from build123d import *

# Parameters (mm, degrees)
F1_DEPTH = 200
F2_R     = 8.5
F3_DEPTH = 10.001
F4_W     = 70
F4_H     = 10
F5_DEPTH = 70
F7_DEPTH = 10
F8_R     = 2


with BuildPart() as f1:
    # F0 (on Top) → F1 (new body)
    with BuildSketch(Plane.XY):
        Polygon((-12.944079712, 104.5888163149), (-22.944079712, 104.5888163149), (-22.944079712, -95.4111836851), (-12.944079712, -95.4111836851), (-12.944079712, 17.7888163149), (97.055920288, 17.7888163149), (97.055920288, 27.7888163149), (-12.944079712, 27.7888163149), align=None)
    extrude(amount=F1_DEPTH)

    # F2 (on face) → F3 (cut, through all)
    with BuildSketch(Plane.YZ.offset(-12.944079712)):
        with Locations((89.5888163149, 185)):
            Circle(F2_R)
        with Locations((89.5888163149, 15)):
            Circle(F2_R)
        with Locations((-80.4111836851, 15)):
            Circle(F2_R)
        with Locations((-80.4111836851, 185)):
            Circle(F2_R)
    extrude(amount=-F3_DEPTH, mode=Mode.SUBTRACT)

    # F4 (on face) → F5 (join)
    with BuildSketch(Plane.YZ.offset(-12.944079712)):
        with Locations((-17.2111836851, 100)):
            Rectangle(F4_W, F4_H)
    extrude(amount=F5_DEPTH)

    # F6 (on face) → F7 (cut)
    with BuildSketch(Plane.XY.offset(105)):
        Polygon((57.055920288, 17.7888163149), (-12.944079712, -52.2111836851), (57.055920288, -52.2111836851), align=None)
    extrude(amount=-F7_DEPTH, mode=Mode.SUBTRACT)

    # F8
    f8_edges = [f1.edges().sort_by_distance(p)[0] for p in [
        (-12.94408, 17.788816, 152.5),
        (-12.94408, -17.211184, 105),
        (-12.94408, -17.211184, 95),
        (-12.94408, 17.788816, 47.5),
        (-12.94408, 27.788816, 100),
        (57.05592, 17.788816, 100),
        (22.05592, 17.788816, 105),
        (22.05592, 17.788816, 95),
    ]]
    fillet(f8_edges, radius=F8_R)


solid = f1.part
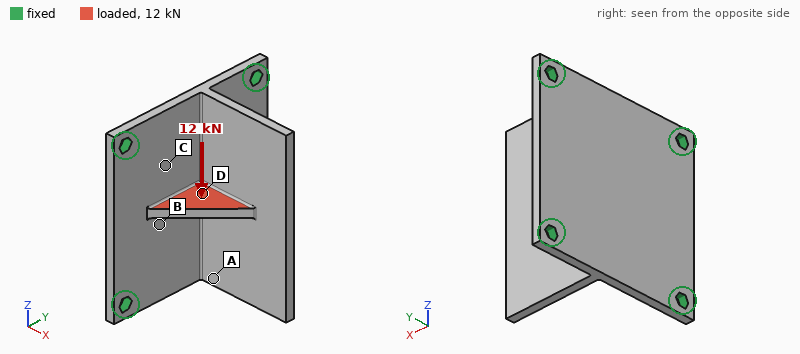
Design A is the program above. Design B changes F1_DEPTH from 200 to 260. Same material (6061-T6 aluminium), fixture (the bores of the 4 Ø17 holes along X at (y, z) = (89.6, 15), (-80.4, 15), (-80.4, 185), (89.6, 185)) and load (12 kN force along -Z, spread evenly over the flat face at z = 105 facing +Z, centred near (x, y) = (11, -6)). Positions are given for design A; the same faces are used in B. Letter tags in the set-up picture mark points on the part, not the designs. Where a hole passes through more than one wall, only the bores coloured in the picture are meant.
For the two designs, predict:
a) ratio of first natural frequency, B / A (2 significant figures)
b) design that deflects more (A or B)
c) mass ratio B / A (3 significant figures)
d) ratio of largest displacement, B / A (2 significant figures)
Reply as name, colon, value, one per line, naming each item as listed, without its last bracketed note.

ratio of first natural frequency, B / A: 0.84
design that deflects more: A
mass ratio B / A: 1.29
ratio of largest displacement, B / A: 0.83
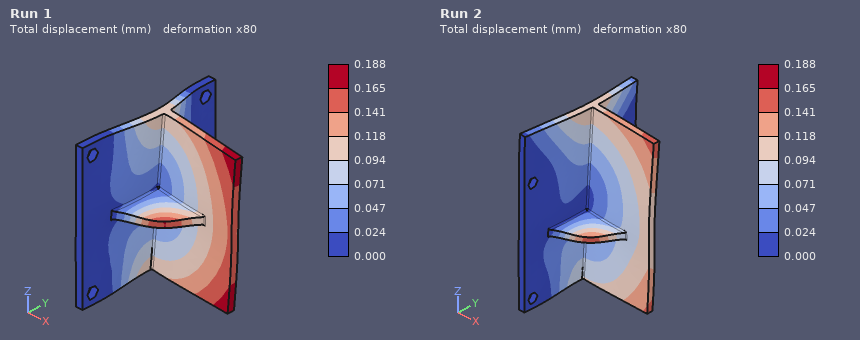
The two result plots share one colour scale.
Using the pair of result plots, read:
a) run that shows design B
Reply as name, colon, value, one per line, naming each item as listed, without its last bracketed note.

run that shows design B: Run 2
